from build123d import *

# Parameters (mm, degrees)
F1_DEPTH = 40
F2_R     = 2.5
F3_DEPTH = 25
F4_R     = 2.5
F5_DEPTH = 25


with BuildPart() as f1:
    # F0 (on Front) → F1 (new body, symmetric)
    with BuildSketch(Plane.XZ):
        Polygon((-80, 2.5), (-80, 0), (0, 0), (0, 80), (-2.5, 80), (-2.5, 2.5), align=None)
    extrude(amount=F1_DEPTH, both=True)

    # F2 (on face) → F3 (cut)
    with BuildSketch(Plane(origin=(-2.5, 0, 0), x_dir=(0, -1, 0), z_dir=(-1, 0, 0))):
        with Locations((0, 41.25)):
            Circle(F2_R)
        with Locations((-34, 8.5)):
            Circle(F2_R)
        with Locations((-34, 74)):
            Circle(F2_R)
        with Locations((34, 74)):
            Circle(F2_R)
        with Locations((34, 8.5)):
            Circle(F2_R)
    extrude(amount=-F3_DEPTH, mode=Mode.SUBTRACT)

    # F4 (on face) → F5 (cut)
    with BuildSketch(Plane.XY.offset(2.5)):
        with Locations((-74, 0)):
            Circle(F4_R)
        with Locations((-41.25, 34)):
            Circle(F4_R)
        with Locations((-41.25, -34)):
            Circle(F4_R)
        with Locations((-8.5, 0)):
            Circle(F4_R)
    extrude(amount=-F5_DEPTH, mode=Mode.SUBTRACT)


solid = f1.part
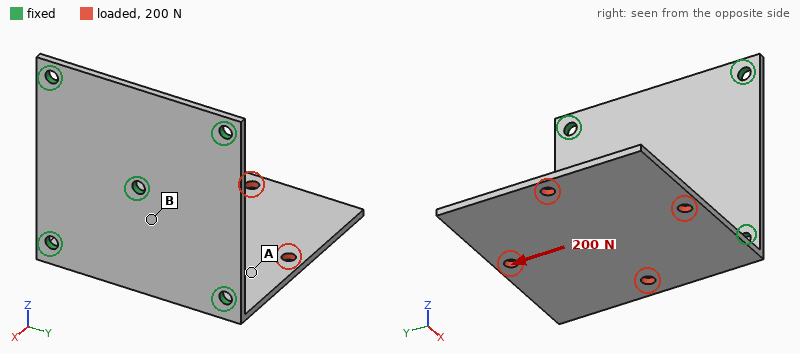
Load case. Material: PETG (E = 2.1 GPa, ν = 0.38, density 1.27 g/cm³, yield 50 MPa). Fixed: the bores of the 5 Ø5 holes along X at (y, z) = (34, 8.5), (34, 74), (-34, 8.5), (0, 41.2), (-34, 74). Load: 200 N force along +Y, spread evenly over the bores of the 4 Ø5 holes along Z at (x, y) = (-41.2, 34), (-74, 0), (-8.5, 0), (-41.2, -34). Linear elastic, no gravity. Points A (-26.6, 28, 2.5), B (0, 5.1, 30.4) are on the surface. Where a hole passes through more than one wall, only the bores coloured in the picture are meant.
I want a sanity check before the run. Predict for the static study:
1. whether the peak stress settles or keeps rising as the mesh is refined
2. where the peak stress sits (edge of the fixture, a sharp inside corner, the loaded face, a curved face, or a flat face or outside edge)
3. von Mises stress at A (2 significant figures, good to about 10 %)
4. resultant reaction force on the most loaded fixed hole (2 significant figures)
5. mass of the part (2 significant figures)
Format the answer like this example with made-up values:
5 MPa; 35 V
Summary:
keeps rising; edge of the fixture; 2.8 MPa; 150 N; 39 g
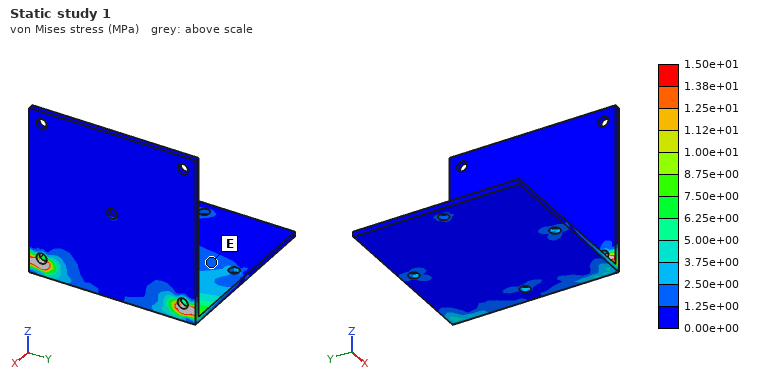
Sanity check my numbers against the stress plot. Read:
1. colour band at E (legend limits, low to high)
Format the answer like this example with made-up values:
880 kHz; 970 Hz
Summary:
1.25e+00 to 2.50e+00 MPa
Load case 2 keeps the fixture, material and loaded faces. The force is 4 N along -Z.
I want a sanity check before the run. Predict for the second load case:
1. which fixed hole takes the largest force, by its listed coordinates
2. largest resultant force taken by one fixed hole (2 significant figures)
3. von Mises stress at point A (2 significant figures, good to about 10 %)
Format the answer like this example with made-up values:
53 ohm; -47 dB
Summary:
(0, 41.2); 2.9 N; 0.84 MPa
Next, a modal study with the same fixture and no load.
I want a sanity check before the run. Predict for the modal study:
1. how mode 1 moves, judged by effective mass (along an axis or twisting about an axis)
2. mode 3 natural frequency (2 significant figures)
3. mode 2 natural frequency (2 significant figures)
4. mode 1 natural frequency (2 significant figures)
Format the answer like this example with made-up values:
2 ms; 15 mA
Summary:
along Z; 470 Hz; 190 Hz; 75 Hz
